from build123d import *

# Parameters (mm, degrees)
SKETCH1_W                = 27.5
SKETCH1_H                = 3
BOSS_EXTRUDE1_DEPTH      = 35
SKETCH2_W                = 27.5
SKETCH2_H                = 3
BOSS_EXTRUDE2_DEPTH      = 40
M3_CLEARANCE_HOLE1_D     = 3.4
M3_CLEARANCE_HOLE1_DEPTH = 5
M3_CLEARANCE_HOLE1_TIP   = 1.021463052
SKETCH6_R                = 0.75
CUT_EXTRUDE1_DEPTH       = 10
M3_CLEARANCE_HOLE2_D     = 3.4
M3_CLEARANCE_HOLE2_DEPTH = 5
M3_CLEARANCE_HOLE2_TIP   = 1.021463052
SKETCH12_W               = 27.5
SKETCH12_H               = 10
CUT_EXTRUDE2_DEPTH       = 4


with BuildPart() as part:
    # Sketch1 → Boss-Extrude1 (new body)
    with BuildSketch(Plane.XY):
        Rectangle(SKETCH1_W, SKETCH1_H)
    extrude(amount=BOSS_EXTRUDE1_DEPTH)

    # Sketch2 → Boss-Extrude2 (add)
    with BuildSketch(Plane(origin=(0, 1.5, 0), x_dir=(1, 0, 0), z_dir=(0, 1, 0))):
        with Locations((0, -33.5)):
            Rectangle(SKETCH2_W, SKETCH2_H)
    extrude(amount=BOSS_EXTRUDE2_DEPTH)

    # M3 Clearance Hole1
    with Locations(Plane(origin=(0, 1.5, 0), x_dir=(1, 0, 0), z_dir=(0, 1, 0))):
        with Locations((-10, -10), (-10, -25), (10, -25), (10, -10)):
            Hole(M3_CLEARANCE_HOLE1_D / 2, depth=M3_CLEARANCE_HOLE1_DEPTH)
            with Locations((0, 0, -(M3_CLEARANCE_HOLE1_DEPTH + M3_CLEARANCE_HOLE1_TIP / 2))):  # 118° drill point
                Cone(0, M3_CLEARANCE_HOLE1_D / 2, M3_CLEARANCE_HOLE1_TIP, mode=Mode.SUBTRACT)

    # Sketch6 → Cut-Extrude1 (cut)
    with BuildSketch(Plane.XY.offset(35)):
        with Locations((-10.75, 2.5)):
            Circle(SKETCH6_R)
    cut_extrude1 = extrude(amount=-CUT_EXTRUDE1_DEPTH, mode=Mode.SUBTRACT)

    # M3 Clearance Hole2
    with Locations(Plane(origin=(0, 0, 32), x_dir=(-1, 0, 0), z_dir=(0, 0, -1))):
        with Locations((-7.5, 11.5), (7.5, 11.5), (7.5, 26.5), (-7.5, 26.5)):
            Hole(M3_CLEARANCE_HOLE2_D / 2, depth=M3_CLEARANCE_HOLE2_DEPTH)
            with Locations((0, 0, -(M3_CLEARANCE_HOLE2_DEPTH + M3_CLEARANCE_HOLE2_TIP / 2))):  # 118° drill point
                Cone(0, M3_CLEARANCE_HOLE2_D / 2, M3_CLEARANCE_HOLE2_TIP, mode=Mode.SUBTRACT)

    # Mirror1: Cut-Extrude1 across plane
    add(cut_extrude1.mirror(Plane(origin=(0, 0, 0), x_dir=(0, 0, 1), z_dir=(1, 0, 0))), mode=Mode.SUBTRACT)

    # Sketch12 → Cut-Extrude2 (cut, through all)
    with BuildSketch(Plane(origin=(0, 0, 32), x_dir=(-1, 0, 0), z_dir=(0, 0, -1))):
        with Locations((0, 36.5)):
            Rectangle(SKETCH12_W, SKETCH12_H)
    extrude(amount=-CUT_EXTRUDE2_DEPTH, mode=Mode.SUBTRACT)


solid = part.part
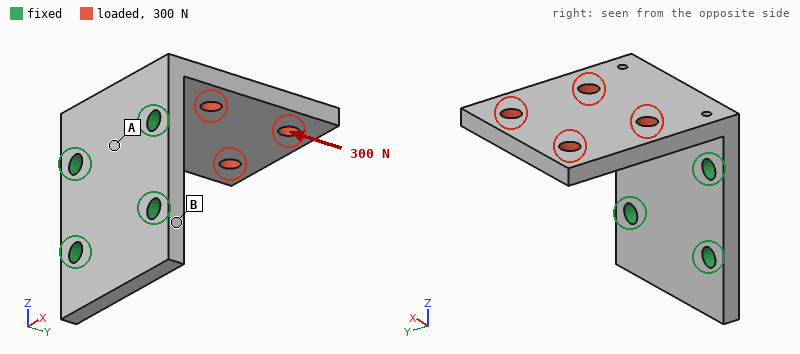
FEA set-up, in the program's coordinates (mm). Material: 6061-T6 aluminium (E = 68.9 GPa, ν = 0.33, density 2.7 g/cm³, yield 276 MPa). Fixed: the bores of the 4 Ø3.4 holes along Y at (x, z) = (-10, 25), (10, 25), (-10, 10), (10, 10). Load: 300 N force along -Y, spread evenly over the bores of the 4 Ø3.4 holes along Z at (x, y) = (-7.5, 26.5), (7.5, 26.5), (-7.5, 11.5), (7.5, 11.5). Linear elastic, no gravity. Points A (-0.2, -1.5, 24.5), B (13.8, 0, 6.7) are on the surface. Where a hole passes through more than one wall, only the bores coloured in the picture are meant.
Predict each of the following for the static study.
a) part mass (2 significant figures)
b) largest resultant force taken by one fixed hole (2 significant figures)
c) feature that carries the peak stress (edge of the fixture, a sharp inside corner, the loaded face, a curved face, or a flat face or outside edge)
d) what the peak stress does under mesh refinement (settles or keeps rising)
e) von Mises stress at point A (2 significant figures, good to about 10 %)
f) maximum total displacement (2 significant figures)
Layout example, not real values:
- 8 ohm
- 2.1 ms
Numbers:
- 14 g
- 170 N
- edge of the fixture
- keeps rising
- 17 MPa
- 75 µm
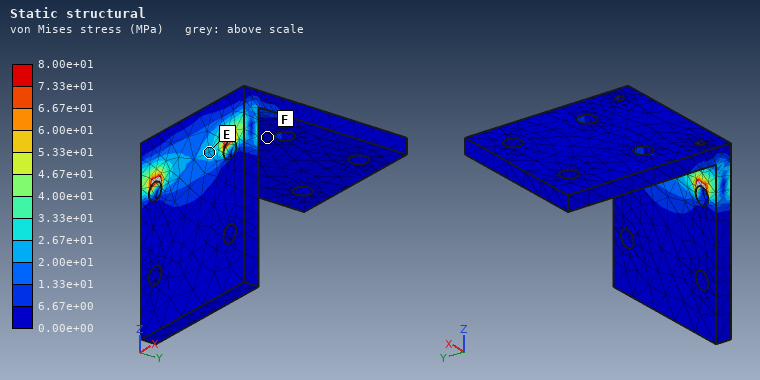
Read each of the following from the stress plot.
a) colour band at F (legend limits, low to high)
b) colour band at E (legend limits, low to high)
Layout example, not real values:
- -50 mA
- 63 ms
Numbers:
- 0.00e+00 to 6.67e+00 MPa
- 2.00e+01 to 2.67e+01 MPa
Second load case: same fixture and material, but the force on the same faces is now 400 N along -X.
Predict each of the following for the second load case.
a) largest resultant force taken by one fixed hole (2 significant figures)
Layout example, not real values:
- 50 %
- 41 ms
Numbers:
- 450 N
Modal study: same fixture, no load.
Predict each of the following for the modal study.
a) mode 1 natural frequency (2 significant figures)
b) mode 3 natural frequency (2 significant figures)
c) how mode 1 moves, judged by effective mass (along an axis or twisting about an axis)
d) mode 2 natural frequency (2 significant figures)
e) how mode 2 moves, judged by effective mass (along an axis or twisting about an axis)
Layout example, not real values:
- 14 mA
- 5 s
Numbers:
- 1800 Hz
- 6700 Hz
- along Z
- 5000 Hz
- along X
